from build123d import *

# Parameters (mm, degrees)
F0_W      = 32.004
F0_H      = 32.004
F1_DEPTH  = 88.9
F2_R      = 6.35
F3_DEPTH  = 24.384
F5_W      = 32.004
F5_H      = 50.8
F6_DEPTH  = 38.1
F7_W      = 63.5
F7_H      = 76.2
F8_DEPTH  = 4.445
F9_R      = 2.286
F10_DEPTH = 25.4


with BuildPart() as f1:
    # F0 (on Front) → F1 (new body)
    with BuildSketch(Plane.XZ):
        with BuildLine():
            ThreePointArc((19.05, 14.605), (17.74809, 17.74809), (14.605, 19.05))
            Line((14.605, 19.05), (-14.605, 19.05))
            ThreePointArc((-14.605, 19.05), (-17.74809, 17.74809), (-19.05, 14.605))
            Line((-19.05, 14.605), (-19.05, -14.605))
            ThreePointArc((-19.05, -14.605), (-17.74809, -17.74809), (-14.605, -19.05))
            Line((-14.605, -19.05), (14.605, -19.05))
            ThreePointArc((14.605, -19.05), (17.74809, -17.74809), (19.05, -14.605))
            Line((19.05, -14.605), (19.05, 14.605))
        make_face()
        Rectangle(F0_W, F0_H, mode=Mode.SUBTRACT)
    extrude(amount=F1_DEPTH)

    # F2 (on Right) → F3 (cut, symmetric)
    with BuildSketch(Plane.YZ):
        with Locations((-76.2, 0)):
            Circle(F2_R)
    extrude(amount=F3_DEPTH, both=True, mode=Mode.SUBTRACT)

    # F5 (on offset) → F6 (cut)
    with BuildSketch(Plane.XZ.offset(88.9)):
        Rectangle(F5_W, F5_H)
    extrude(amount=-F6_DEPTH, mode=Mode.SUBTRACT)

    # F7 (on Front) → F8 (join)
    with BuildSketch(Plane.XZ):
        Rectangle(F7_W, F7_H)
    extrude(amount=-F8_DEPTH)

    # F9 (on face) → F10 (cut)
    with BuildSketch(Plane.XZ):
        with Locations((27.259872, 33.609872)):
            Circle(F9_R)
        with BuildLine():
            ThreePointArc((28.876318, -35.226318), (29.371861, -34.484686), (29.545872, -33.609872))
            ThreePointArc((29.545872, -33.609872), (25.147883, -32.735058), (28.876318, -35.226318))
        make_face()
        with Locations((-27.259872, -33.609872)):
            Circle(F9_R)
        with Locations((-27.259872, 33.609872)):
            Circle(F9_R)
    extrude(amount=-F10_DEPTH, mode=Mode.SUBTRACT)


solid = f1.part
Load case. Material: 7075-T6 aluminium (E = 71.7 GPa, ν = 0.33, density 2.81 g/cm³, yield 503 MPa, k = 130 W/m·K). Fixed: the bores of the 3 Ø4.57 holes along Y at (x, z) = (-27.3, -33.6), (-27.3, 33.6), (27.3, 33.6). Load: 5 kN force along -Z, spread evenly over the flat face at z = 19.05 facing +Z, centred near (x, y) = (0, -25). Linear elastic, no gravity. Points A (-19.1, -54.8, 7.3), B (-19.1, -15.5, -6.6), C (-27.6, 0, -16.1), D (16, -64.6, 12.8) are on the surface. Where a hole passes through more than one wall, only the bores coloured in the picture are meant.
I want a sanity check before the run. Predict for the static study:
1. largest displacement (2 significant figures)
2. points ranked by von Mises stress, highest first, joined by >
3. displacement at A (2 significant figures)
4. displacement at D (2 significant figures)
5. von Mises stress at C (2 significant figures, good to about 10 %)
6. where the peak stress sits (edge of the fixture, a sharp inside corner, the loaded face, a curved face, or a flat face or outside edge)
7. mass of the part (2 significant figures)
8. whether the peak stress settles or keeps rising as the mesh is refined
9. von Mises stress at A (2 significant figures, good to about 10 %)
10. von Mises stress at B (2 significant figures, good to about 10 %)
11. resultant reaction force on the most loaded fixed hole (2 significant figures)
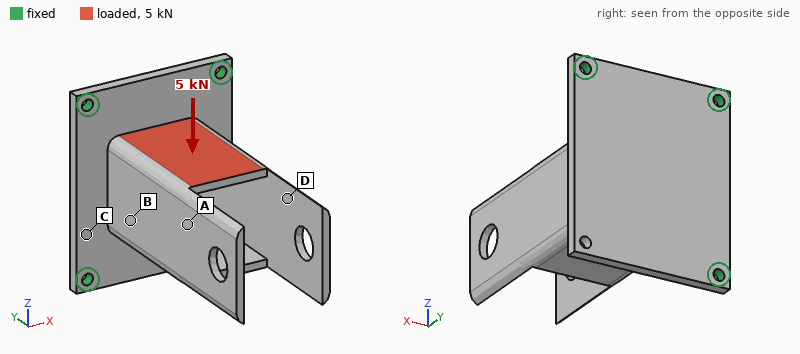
1.3 mm
C > B > A > D
0.53 mm
0.85 mm
110 MPa
edge of the fixture
140 g
keeps rising
46 MPa
73 MPa
2.9 kN
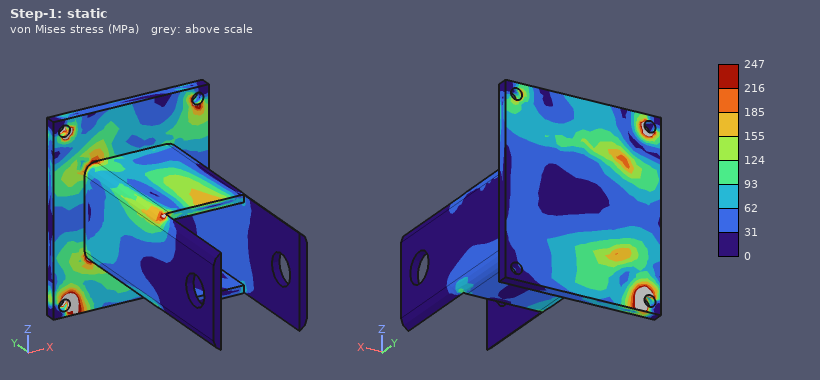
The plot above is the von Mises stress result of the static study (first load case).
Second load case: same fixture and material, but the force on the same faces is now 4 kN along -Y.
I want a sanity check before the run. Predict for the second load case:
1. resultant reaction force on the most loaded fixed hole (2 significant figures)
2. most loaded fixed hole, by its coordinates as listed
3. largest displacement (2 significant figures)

2.0 kN
(27.3, 33.6)
0.25 mm
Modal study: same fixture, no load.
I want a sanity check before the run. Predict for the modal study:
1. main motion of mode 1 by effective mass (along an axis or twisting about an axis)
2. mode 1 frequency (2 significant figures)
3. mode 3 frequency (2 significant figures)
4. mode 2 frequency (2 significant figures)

along X
850 Hz
1400 Hz
1300 Hz
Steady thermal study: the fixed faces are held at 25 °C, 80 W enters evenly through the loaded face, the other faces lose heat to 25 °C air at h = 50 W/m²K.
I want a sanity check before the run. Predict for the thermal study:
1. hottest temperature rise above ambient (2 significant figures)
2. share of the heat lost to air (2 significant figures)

68 K
50 %
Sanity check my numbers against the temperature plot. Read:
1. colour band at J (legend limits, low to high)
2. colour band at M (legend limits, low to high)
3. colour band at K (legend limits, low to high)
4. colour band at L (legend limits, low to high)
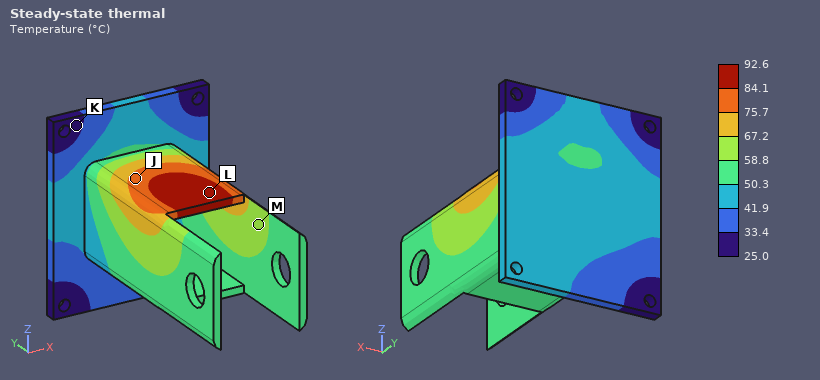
75.7 to 84.1 °C
58.8 to 67.2 °C
25.0 to 33.4 °C
84.1 to 92.6 °C
